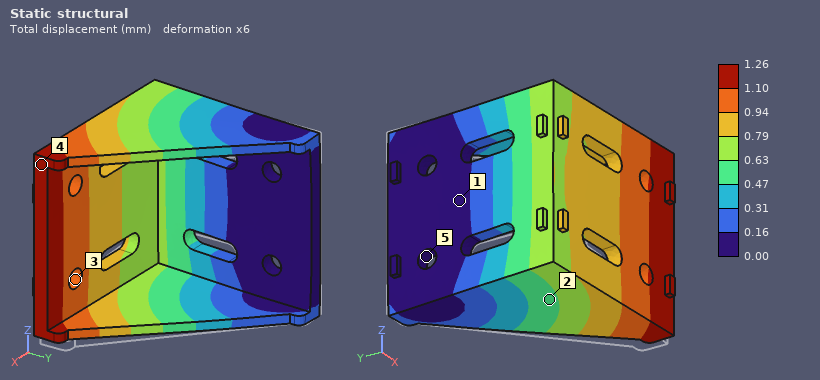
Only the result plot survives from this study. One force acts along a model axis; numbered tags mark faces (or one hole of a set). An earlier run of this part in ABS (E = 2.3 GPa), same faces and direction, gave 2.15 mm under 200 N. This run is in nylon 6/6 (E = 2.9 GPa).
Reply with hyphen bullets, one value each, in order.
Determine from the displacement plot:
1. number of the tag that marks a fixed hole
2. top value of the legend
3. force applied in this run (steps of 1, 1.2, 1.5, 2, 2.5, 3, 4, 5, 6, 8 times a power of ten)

- 5
- 1.26 mm
- 150 N
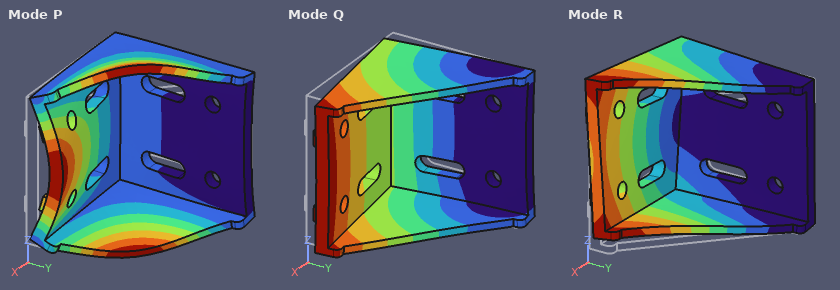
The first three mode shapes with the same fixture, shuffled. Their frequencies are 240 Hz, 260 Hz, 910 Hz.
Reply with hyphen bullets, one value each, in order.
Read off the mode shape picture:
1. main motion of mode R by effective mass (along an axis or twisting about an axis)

- along Z
